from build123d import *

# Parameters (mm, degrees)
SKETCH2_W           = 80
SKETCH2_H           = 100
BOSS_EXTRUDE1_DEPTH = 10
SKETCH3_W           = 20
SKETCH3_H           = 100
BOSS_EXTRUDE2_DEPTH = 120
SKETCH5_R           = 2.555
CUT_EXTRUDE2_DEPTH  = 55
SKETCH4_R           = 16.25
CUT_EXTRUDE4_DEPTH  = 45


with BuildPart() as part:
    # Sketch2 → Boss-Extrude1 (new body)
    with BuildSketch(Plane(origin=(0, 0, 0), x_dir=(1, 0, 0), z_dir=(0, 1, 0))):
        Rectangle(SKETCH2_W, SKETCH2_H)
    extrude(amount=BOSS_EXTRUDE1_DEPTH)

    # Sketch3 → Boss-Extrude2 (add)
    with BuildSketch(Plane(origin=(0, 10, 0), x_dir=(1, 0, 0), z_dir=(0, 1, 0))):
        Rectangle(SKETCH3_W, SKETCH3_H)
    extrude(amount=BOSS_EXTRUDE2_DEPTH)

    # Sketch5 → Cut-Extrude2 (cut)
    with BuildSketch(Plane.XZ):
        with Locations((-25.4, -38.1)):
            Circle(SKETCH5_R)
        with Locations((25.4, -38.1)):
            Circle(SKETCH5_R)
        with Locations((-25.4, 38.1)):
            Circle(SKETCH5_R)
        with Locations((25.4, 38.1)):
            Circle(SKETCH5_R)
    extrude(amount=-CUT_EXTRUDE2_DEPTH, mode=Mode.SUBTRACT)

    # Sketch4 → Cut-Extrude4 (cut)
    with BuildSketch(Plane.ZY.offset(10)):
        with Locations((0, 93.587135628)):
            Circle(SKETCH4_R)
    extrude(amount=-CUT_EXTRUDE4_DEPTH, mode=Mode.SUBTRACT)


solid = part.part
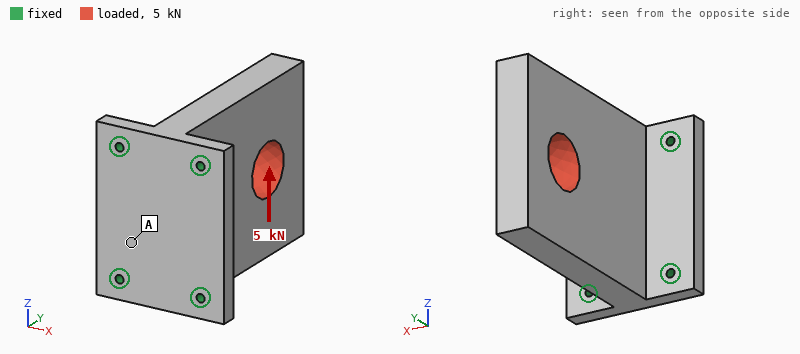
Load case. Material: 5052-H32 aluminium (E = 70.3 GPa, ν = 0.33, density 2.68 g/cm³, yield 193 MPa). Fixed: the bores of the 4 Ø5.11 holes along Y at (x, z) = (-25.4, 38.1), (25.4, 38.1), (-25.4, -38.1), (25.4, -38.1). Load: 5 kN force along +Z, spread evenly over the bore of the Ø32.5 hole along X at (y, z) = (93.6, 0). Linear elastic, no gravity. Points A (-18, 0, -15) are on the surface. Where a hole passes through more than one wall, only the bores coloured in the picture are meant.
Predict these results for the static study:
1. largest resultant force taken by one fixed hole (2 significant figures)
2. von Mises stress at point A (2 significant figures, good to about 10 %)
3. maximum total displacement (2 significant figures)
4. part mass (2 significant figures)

3.3 kN
7.8 MPa
0.10 mm
810 g
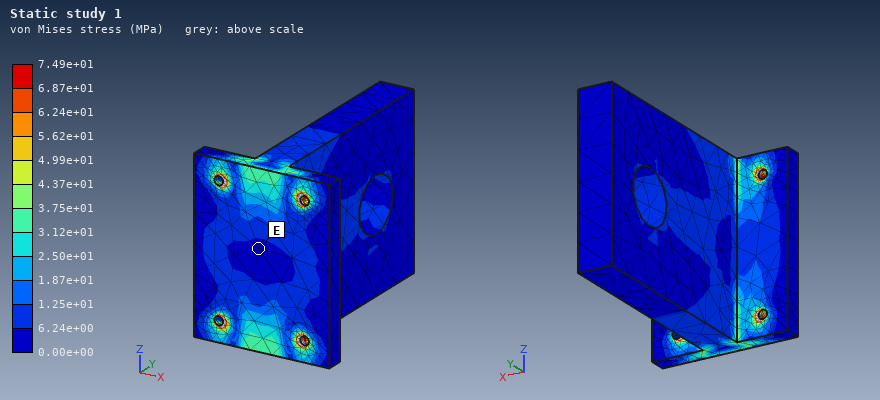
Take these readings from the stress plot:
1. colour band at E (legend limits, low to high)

0.00e+00 to 6.24e+00 MPa
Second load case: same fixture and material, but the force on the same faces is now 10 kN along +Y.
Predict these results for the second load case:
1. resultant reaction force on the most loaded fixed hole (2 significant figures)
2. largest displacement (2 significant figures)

2.6 kN
29 µm
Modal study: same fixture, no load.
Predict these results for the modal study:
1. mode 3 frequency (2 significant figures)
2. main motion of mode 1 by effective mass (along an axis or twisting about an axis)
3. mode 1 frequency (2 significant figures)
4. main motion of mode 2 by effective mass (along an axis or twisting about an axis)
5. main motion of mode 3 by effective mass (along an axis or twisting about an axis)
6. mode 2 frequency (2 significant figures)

2500 Hz
along X
890 Hz
along Z
twisting about Y
2000 Hz
